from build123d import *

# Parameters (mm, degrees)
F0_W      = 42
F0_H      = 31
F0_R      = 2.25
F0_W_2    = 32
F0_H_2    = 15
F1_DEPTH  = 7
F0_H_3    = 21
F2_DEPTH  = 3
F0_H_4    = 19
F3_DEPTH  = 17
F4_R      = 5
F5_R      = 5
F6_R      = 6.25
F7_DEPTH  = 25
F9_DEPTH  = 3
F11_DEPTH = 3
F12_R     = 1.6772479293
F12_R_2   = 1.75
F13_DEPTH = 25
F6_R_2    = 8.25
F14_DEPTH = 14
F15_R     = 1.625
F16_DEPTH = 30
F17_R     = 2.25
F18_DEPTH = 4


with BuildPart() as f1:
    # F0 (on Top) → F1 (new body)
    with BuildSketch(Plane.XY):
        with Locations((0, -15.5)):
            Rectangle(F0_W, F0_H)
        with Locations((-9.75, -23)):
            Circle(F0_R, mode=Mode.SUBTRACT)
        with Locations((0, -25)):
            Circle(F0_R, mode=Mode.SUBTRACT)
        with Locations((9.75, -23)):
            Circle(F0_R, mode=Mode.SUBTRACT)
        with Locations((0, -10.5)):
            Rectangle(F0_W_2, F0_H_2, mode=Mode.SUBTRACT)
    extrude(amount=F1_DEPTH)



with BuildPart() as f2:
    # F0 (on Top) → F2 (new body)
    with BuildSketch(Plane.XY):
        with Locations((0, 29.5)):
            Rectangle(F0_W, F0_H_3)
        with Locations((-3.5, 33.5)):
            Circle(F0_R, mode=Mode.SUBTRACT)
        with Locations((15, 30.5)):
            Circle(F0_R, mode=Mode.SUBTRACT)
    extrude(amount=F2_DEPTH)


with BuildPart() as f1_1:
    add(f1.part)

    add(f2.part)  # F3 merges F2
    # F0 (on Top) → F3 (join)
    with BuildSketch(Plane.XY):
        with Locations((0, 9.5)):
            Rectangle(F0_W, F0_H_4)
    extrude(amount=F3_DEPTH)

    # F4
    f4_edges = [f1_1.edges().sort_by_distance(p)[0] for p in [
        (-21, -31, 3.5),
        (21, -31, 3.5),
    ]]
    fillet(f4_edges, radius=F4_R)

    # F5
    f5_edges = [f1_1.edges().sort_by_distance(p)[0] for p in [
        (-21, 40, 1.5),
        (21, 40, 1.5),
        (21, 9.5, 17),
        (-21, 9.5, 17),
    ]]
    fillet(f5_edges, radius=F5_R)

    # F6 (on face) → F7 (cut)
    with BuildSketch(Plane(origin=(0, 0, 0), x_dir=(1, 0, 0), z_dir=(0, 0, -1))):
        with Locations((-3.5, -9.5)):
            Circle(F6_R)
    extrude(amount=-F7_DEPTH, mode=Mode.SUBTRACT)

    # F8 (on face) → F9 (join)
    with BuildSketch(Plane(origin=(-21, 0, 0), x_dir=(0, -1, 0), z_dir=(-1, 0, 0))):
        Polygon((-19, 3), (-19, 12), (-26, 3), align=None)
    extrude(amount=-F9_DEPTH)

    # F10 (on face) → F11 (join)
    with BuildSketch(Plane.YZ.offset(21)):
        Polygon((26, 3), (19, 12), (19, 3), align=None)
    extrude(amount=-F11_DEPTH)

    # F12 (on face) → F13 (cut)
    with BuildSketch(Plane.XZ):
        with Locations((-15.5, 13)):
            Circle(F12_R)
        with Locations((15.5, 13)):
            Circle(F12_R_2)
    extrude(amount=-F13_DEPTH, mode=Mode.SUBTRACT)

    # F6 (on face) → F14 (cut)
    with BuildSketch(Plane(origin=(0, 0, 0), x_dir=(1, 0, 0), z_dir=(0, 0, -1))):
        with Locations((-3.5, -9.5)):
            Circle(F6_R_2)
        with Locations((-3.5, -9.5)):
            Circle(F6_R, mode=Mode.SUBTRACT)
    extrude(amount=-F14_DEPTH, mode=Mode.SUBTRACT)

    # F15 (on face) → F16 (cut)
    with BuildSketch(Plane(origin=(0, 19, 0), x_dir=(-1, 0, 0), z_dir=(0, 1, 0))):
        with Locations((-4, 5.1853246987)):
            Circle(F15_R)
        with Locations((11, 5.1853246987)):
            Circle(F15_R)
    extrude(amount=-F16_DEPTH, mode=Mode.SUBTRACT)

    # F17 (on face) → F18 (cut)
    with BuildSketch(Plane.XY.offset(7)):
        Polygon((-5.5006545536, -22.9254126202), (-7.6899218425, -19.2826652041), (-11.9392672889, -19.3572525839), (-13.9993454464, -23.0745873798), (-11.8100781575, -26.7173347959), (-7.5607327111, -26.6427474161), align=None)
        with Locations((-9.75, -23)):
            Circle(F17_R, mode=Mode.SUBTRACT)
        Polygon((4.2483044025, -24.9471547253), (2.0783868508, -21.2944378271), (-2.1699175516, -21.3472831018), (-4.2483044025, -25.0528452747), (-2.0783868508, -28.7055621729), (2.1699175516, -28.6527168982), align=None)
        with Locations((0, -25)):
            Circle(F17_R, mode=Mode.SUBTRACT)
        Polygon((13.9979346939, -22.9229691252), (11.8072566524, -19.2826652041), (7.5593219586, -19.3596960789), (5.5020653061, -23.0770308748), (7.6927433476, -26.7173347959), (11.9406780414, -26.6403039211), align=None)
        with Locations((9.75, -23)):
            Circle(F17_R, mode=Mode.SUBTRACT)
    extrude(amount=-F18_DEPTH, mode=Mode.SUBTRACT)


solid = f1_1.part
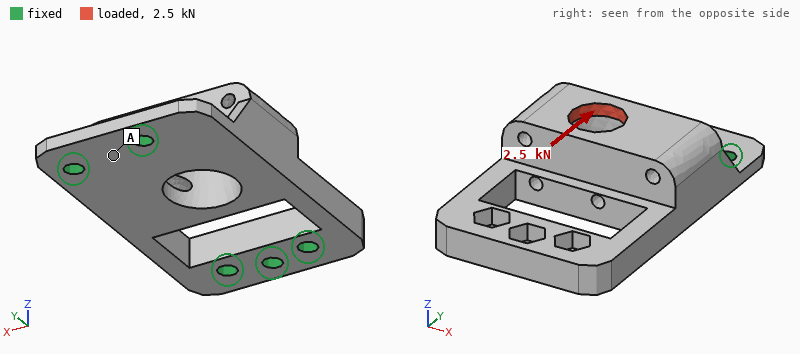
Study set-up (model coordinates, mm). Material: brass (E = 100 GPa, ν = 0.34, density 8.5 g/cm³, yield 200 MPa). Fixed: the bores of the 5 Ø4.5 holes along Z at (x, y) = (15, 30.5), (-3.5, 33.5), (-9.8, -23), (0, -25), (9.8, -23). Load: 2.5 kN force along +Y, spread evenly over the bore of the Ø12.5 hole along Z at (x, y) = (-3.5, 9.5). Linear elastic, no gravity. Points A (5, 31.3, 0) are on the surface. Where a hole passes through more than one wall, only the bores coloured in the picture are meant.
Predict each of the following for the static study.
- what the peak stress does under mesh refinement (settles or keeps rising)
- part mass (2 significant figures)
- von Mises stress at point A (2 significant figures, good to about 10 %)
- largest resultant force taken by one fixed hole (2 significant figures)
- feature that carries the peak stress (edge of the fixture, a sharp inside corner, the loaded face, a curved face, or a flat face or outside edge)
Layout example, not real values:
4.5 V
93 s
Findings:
keeps rising
150 g
15 MPa
980 N
edge of the fixture
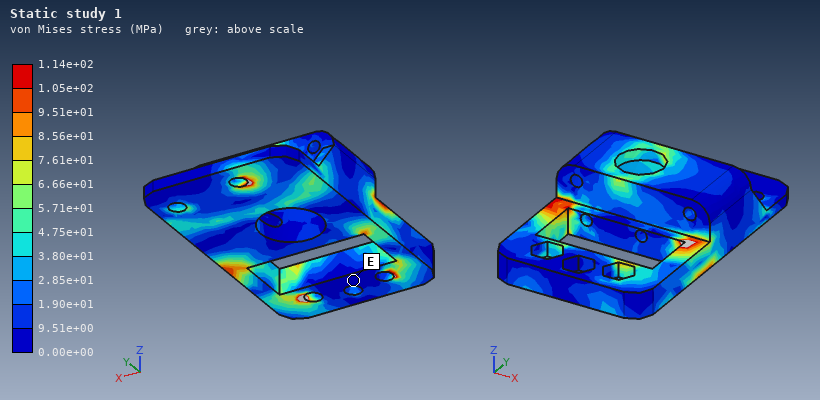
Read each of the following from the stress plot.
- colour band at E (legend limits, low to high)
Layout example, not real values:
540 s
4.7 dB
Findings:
0.00e+00 to 9.51e+00 MPa
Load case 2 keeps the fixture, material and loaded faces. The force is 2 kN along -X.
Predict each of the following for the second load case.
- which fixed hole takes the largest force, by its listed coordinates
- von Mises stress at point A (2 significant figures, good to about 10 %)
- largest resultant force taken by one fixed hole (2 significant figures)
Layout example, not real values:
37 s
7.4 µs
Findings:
(15, 30.5)
17 MPa
1.6 kN
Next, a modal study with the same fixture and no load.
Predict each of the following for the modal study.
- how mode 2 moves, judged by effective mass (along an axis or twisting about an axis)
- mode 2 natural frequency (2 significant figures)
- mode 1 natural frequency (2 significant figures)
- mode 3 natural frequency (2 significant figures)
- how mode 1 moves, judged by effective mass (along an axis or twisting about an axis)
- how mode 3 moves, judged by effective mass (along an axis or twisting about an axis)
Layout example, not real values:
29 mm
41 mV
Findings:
along Z
3700 Hz
2800 Hz
6500 Hz
along Z
along X
